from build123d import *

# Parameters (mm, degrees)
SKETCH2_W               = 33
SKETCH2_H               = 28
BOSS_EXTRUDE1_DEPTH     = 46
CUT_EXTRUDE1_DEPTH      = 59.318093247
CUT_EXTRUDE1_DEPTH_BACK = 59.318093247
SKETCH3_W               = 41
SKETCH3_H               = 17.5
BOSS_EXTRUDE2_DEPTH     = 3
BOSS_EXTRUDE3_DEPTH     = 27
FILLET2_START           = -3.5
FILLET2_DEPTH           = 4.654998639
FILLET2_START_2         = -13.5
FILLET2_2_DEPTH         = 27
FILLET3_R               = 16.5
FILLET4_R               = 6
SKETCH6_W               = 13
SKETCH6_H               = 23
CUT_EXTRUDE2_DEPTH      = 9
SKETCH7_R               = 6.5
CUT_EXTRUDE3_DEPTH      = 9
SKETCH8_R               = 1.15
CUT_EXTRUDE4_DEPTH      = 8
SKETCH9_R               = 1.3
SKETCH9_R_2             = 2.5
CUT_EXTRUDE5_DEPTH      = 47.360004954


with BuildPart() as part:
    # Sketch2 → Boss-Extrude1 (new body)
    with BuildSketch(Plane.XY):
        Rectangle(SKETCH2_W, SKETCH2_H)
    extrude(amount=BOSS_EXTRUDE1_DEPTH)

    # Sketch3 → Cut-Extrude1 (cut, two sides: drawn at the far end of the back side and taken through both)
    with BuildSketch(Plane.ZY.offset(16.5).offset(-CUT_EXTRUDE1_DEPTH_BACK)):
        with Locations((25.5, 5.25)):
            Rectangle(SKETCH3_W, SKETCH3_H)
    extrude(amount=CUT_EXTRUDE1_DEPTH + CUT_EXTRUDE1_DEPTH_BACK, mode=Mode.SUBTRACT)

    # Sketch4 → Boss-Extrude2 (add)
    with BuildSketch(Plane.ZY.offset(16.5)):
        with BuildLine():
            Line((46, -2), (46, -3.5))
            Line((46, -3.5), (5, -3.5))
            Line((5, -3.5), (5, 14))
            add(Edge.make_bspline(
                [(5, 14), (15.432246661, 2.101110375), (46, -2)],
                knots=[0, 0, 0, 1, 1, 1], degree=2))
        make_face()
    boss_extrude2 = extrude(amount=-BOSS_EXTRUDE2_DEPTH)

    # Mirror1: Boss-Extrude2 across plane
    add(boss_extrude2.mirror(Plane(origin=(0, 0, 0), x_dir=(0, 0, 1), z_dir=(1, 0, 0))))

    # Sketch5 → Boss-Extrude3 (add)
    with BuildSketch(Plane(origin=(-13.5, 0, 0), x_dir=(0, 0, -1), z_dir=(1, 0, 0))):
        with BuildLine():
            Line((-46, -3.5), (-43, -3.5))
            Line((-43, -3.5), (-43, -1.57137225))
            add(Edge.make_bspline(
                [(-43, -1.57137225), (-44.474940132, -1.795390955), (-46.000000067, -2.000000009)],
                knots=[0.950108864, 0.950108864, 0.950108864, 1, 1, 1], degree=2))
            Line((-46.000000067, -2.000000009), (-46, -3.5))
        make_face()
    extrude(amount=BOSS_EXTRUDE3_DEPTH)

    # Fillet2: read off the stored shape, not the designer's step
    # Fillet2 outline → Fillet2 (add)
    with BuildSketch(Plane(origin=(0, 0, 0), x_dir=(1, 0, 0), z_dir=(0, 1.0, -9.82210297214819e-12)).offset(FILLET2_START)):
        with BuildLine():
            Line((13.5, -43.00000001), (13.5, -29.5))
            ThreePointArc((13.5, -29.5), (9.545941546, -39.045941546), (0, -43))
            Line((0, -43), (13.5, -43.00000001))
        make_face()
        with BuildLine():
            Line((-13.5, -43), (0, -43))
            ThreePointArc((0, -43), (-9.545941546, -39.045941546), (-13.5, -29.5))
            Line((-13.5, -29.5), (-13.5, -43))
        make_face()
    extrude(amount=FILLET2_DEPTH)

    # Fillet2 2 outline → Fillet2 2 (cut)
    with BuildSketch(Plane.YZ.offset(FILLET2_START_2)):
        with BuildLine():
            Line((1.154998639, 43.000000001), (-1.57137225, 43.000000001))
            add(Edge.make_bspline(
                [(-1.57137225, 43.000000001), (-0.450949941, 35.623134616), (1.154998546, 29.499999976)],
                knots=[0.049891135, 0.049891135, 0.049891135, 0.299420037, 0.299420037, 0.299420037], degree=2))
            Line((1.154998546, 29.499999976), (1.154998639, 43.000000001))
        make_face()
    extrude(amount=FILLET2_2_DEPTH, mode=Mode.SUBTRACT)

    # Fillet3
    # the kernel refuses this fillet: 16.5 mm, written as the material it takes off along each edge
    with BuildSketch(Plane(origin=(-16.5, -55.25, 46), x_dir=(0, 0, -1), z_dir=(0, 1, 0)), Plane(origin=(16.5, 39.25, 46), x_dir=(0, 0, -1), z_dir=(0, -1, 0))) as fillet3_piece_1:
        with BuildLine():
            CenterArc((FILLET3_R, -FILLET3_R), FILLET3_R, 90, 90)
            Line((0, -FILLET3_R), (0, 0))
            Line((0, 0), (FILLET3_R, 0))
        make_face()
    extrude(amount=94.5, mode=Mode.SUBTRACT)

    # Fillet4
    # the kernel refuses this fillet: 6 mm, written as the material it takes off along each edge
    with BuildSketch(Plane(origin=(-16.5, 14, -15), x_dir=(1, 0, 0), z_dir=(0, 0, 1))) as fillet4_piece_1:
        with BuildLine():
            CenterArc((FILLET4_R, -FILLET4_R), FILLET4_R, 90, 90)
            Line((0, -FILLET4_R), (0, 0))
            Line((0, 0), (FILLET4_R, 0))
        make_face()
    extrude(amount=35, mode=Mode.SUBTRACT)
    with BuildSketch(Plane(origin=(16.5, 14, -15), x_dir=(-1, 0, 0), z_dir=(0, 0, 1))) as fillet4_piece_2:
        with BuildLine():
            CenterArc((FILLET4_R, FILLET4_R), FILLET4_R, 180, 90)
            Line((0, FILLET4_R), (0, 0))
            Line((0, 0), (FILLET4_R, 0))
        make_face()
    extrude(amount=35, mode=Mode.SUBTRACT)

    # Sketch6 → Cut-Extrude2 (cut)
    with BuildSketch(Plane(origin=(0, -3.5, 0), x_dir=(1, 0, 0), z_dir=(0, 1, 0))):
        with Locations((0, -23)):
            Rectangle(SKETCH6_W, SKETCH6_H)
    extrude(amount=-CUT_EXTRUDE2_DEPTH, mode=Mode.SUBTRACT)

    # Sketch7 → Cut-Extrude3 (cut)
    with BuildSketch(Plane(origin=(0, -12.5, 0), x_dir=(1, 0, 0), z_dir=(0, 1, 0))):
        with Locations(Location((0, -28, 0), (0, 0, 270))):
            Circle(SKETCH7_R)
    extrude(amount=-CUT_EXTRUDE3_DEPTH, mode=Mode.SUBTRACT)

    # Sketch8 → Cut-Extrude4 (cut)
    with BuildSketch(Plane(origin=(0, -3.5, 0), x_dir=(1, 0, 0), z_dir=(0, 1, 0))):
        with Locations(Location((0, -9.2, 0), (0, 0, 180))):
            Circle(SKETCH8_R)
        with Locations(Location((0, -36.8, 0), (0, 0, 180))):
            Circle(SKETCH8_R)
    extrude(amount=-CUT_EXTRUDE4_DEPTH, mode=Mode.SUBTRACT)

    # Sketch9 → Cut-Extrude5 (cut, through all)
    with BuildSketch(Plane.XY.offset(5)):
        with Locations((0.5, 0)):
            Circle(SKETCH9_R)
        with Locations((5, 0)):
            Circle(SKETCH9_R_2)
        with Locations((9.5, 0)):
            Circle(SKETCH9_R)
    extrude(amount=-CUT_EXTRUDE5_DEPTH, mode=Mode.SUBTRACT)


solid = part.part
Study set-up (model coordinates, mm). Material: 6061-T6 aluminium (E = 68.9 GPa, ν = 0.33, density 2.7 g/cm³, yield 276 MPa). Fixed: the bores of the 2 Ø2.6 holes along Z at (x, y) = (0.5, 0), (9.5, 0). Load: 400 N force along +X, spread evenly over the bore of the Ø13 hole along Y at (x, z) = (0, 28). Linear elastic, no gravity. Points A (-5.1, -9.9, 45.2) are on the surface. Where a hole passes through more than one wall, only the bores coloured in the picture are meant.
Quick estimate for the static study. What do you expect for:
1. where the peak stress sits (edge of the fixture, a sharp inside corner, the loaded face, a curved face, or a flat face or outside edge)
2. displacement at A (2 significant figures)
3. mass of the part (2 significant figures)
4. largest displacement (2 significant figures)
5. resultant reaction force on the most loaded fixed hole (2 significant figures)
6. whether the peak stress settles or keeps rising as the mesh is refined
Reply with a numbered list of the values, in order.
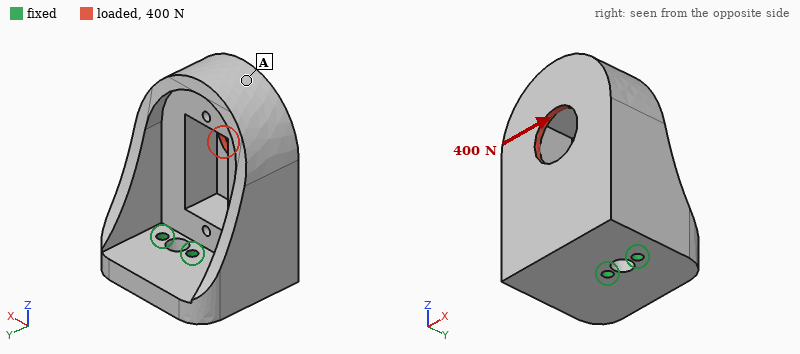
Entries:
1. edge of the fixture
2. 43 µm
3. 44 g
4. 44 µm
5. 860 N
6. keeps rising
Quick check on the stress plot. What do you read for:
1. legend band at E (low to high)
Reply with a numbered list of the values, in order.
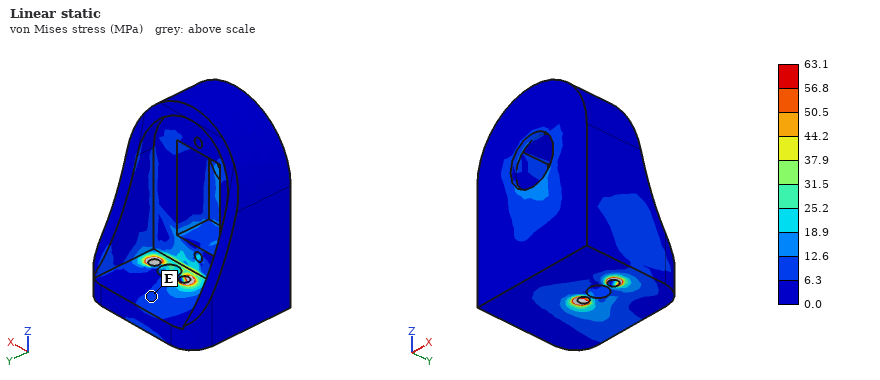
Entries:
1. 6.3 to 12.6 MPa
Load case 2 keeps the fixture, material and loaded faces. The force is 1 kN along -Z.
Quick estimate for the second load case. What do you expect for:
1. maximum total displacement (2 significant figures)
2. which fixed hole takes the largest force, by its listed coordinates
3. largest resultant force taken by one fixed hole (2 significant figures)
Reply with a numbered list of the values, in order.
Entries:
1. 0.12 mm
2. (0.5, 0)
3. 820 N
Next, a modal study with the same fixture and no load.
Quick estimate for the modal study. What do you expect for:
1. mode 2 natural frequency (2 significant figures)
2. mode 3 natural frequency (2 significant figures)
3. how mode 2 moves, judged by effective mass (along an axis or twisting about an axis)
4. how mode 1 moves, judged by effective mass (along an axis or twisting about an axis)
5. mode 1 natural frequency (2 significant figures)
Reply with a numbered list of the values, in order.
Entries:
1. 3200 Hz
2. 7500 Hz
3. along X
4. along Y
5. 2300 Hz
